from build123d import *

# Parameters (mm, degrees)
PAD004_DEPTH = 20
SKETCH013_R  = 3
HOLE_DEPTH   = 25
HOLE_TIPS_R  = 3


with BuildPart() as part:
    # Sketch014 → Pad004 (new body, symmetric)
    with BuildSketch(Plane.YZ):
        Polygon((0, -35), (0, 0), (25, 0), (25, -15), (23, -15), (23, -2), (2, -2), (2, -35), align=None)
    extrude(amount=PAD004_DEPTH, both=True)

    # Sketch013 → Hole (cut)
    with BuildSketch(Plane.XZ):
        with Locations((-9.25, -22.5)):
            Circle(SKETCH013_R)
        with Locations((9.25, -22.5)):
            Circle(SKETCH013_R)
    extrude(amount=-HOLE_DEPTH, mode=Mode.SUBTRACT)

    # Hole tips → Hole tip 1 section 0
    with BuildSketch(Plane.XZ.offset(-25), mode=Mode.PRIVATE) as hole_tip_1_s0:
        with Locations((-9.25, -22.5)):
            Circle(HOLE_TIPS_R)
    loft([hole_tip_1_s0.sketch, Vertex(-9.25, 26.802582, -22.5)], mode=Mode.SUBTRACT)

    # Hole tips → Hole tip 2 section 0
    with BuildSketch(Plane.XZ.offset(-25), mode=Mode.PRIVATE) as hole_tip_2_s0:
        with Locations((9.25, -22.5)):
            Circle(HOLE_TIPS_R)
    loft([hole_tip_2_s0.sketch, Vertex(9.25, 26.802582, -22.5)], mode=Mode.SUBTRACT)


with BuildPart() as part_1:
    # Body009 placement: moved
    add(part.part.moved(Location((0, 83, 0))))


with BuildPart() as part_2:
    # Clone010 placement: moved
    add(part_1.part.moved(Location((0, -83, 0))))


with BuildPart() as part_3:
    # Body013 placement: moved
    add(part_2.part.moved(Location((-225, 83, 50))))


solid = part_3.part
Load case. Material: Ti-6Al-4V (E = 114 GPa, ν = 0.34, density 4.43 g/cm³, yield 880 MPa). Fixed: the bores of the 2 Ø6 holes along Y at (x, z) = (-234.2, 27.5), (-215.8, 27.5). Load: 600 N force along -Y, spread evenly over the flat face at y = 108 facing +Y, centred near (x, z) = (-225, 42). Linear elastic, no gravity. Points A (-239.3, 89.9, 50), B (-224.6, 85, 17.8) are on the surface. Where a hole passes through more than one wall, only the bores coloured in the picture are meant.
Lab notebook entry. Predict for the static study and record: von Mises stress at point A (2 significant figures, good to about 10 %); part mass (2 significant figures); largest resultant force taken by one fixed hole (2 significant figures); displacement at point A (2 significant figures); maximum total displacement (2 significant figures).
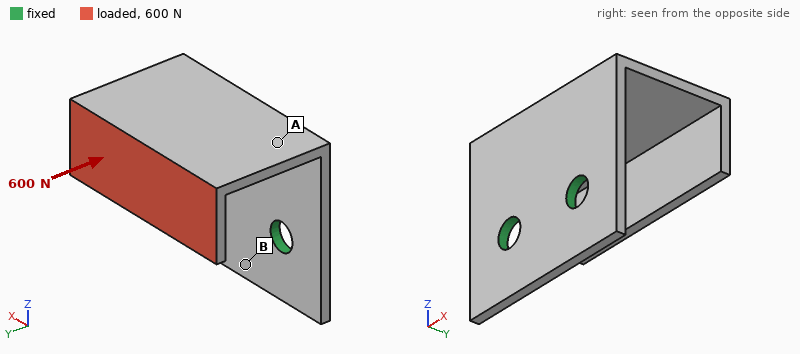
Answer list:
120 MPa
25 g
300 N
0.26 mm
0.48 mm
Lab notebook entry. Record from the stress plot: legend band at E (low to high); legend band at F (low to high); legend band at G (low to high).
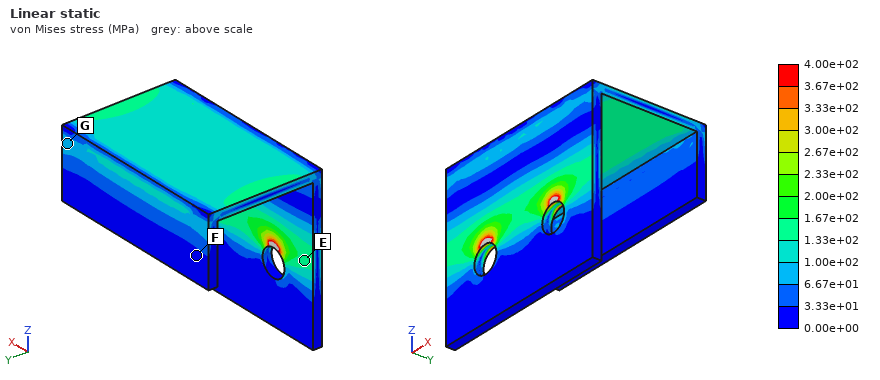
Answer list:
1.33e+02 to 1.67e+02 MPa
0.00e+00 to 3.33e+01 MPa
6.67e+01 to 1.00e+02 MPa
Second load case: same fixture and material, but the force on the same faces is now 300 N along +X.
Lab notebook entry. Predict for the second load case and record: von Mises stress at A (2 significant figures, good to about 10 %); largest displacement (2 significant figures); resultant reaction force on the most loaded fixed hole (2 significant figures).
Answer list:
93 MPa
0.64 mm
370 N
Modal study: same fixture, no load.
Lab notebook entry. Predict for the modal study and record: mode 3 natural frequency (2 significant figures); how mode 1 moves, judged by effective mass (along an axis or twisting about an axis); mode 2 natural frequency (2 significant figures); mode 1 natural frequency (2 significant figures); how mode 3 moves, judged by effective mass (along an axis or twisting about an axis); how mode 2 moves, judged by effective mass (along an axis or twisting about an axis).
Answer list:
2100 Hz
along Z
1300 Hz
820 Hz
along Y
along X
